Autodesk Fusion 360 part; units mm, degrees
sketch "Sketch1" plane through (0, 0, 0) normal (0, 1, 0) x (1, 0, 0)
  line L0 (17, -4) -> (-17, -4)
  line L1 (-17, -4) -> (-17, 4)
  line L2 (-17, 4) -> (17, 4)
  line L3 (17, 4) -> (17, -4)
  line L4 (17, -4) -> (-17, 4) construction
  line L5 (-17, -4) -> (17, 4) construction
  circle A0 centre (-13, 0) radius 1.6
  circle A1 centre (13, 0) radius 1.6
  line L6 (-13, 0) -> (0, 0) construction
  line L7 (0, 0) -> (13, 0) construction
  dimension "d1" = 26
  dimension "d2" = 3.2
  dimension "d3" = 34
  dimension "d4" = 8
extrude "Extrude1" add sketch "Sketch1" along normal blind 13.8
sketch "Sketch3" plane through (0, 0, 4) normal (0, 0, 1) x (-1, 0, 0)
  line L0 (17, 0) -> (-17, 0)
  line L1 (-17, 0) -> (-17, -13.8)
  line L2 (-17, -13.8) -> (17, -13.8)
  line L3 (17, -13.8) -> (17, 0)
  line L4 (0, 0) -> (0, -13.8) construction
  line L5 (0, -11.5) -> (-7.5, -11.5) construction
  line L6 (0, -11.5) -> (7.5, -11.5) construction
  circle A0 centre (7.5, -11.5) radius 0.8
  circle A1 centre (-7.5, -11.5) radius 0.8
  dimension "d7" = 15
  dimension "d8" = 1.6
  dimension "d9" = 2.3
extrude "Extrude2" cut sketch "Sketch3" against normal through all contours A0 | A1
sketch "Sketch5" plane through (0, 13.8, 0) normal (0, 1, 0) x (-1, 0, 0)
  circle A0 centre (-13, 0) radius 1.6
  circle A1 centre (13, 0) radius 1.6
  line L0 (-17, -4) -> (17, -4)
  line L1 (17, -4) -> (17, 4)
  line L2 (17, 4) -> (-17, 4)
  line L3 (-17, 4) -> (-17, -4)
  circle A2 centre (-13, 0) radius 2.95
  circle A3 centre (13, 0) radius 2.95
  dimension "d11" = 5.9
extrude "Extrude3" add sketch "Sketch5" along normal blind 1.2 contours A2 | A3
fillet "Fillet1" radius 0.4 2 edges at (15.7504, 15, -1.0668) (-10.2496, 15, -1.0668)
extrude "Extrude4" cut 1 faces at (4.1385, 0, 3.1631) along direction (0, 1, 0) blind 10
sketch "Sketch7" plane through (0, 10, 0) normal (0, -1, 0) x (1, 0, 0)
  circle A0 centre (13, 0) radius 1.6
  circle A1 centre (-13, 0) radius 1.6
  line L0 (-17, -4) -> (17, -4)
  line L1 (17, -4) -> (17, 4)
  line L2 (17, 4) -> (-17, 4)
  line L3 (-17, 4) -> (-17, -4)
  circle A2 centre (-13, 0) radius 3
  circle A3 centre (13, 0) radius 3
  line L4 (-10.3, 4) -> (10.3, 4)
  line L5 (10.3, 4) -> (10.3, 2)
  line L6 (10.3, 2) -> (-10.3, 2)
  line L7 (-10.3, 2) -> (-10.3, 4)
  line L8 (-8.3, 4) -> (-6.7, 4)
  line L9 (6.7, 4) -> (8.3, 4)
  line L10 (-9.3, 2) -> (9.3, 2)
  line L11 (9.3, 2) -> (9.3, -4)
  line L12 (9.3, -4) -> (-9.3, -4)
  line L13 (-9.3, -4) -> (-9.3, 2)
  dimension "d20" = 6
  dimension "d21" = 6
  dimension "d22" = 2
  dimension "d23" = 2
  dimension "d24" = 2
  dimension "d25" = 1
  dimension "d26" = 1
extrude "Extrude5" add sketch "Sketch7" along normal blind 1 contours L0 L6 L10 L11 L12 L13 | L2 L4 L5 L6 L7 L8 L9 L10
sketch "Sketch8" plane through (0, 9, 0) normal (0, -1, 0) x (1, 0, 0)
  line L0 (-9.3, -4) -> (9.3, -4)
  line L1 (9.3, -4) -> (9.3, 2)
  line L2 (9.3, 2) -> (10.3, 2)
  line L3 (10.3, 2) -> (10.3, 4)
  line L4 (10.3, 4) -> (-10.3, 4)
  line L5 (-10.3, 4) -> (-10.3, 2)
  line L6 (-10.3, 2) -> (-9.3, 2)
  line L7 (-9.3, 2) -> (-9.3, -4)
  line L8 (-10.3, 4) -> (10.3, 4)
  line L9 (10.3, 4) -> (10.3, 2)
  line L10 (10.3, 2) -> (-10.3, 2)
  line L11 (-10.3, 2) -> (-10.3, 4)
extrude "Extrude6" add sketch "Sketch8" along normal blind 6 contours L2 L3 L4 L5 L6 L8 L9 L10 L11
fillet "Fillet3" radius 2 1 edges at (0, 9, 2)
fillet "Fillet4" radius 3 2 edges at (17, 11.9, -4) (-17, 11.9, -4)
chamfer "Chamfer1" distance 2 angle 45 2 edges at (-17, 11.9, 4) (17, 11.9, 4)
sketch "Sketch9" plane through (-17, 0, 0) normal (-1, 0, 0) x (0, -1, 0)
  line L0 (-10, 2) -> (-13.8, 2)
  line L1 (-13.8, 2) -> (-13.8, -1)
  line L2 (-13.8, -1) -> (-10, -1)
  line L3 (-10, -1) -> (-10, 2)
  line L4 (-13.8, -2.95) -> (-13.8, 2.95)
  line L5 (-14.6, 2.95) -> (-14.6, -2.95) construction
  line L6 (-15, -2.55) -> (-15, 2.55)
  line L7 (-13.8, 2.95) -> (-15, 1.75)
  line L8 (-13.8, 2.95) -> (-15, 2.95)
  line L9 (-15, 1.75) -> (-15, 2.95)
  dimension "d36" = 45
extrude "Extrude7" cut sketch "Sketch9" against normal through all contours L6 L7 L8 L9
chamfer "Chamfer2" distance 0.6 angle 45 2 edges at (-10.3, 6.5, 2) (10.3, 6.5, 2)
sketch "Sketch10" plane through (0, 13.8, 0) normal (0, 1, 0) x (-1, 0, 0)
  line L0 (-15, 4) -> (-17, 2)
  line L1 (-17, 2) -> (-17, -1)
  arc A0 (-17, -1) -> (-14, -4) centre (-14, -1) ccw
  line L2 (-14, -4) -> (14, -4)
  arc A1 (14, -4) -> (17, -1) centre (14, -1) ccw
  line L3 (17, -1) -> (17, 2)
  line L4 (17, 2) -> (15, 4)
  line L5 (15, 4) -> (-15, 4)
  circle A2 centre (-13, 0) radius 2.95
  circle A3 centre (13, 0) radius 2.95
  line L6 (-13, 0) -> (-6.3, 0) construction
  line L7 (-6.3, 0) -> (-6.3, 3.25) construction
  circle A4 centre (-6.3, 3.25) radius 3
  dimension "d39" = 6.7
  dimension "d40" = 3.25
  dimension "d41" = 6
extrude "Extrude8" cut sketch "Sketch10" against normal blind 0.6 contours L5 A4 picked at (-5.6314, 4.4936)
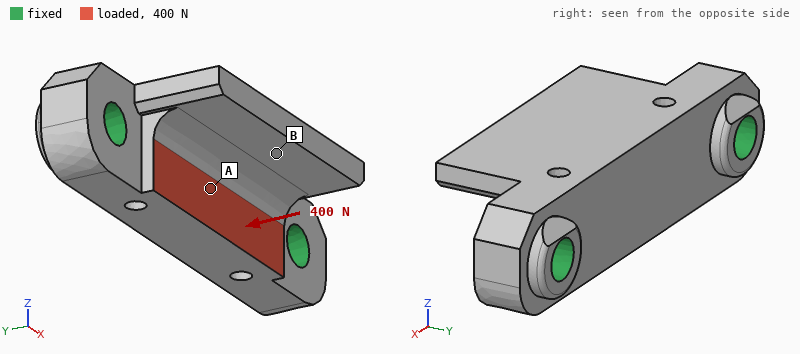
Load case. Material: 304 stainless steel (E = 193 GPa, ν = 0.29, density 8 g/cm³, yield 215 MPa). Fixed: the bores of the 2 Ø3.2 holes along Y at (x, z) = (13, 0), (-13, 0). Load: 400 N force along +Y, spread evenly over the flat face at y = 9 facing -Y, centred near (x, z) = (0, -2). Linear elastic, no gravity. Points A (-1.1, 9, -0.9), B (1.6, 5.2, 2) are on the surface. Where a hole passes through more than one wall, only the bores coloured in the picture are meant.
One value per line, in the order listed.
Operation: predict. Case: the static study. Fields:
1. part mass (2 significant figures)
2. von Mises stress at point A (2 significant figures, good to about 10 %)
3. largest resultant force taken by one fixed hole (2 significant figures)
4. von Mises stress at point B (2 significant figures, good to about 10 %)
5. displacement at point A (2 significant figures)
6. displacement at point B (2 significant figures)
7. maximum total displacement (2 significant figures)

11 g
13 MPa
220 N
5.6 MPa
2.1 µm
1.9 µm
3.1 µm
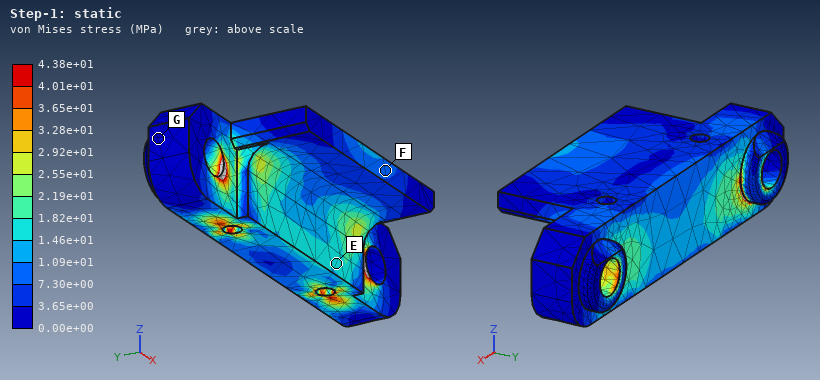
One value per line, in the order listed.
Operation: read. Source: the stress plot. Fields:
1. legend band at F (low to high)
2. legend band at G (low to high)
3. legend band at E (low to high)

7.30e+00 to 1.09e+01 MPa
0.00e+00 to 3.65e+00 MPa
1.46e+01 to 1.82e+01 MPa
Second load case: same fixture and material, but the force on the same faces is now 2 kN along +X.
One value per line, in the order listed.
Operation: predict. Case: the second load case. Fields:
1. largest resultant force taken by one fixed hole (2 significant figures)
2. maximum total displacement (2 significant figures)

1.0 kN
2.5 µm
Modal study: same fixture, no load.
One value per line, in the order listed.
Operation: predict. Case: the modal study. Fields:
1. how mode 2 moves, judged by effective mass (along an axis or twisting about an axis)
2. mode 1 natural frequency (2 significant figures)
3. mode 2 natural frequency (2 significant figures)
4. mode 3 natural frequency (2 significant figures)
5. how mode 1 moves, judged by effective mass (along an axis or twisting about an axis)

along Y
22 kHz
33 kHz
39 kHz
along Z
